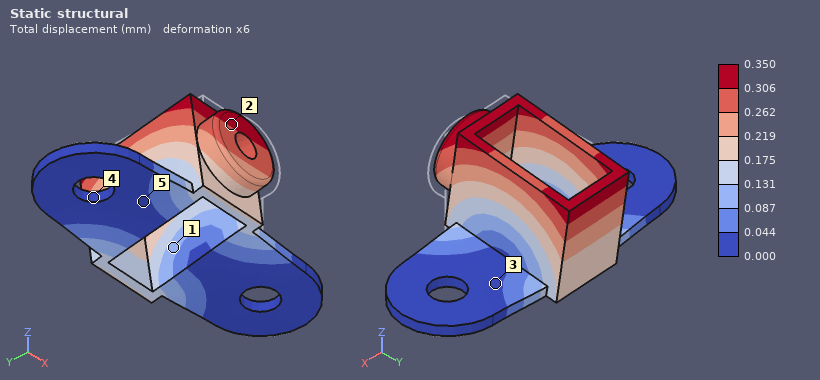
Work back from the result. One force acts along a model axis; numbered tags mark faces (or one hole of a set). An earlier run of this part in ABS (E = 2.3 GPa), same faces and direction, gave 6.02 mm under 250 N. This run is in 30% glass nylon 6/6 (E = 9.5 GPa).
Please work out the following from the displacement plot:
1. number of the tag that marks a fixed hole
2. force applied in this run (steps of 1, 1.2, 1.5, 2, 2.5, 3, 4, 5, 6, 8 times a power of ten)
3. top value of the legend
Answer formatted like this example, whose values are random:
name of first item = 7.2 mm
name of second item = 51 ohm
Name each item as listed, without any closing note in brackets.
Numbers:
number of the tag that marks a fixed hole = 4
force applied in this run = 60 N
top value of the legend = 0.350 mm
